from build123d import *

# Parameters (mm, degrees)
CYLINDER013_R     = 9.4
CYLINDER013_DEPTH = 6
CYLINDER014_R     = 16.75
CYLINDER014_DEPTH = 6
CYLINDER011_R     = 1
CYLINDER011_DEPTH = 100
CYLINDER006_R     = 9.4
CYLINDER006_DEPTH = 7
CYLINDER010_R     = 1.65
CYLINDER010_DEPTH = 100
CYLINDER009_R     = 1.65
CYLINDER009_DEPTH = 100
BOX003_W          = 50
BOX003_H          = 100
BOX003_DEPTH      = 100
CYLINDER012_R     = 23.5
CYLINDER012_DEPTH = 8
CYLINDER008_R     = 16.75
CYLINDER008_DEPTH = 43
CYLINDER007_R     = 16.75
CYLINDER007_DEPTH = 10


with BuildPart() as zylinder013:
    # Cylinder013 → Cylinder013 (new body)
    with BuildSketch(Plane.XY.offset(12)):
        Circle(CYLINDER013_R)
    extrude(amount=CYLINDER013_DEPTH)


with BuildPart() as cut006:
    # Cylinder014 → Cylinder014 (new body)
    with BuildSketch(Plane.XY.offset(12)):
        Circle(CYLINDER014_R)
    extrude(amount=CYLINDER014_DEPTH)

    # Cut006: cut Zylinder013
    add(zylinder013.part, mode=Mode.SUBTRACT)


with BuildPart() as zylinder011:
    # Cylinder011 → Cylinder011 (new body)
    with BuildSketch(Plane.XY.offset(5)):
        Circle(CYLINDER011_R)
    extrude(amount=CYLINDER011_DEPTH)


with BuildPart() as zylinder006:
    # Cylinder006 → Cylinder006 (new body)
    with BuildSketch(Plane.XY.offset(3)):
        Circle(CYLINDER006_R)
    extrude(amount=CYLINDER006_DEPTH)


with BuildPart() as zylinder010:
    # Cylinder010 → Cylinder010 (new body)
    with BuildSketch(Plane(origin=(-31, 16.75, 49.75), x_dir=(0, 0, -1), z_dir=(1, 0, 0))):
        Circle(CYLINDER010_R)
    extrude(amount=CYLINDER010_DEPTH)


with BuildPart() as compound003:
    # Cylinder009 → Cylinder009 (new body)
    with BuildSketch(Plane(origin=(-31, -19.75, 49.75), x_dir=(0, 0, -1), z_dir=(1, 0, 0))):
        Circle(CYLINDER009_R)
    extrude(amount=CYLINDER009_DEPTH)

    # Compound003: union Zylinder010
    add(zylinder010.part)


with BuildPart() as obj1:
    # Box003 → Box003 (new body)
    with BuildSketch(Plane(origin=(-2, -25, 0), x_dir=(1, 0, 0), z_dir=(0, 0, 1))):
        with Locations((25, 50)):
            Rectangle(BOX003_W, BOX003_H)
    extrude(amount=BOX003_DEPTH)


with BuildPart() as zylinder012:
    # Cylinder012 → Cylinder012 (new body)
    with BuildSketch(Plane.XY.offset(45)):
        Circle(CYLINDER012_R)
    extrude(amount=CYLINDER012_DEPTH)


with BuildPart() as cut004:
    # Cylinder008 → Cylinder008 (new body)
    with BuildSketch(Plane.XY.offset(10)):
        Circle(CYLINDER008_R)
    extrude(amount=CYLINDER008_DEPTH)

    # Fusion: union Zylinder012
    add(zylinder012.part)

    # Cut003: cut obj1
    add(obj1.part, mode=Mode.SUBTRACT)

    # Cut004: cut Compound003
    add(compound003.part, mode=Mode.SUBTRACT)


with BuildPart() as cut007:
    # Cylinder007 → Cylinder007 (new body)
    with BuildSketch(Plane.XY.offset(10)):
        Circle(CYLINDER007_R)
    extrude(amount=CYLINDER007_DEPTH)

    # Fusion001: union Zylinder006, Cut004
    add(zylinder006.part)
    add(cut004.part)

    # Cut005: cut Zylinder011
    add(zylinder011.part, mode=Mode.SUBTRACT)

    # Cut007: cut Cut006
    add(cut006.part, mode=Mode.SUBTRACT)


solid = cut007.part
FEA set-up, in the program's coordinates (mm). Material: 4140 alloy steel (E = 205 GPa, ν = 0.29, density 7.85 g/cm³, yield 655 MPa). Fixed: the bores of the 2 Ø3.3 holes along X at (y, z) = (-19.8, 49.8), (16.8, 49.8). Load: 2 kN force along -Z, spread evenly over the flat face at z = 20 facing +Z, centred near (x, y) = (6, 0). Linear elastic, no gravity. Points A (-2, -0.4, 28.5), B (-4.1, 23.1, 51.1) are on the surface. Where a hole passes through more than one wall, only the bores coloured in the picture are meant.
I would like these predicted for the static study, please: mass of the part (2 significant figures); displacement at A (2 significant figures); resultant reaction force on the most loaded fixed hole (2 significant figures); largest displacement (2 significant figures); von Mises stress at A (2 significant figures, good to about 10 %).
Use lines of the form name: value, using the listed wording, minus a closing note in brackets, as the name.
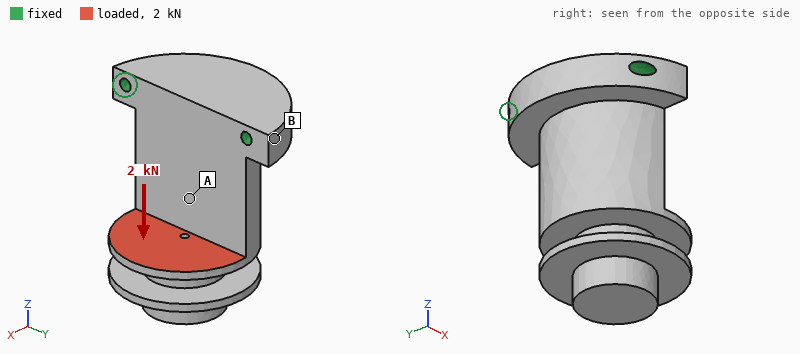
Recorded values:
mass of the part: 180 g
displacement at A: 15 µm
resultant reaction force on the most loaded fixed hole: 1.1 kN
largest displacement: 78 µm
von Mises stress at A: 42 MPa
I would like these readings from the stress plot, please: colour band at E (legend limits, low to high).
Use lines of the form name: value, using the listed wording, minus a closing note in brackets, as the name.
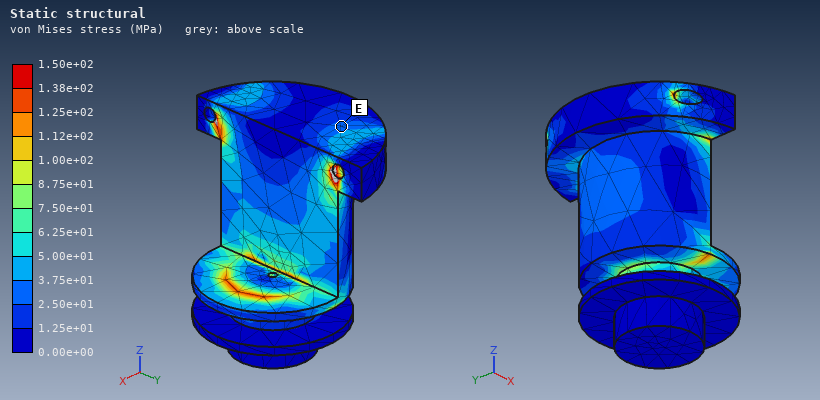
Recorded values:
colour band at E: 2.50e+01 to 3.75e+01 MPa
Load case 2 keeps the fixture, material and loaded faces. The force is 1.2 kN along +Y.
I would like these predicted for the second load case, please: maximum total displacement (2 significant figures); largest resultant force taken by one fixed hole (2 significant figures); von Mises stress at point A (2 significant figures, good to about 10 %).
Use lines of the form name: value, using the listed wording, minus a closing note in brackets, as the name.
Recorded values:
maximum total displacement: 18 µm
largest resultant force taken by one fixed hole: 1.3 kN
von Mises stress at point A: 35 MPa
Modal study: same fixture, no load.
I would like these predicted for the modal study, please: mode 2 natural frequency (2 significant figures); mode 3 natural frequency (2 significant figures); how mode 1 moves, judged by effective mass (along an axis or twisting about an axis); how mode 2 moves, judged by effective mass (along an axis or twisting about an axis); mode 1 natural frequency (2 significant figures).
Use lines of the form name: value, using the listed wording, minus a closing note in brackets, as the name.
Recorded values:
mode 2 natural frequency: 6700 Hz
mode 3 natural frequency: 9700 Hz
how mode 1 moves, judged by effective mass: along X
how mode 2 moves, judged by effective mass: along Y
mode 1 natural frequency: 2900 Hz
